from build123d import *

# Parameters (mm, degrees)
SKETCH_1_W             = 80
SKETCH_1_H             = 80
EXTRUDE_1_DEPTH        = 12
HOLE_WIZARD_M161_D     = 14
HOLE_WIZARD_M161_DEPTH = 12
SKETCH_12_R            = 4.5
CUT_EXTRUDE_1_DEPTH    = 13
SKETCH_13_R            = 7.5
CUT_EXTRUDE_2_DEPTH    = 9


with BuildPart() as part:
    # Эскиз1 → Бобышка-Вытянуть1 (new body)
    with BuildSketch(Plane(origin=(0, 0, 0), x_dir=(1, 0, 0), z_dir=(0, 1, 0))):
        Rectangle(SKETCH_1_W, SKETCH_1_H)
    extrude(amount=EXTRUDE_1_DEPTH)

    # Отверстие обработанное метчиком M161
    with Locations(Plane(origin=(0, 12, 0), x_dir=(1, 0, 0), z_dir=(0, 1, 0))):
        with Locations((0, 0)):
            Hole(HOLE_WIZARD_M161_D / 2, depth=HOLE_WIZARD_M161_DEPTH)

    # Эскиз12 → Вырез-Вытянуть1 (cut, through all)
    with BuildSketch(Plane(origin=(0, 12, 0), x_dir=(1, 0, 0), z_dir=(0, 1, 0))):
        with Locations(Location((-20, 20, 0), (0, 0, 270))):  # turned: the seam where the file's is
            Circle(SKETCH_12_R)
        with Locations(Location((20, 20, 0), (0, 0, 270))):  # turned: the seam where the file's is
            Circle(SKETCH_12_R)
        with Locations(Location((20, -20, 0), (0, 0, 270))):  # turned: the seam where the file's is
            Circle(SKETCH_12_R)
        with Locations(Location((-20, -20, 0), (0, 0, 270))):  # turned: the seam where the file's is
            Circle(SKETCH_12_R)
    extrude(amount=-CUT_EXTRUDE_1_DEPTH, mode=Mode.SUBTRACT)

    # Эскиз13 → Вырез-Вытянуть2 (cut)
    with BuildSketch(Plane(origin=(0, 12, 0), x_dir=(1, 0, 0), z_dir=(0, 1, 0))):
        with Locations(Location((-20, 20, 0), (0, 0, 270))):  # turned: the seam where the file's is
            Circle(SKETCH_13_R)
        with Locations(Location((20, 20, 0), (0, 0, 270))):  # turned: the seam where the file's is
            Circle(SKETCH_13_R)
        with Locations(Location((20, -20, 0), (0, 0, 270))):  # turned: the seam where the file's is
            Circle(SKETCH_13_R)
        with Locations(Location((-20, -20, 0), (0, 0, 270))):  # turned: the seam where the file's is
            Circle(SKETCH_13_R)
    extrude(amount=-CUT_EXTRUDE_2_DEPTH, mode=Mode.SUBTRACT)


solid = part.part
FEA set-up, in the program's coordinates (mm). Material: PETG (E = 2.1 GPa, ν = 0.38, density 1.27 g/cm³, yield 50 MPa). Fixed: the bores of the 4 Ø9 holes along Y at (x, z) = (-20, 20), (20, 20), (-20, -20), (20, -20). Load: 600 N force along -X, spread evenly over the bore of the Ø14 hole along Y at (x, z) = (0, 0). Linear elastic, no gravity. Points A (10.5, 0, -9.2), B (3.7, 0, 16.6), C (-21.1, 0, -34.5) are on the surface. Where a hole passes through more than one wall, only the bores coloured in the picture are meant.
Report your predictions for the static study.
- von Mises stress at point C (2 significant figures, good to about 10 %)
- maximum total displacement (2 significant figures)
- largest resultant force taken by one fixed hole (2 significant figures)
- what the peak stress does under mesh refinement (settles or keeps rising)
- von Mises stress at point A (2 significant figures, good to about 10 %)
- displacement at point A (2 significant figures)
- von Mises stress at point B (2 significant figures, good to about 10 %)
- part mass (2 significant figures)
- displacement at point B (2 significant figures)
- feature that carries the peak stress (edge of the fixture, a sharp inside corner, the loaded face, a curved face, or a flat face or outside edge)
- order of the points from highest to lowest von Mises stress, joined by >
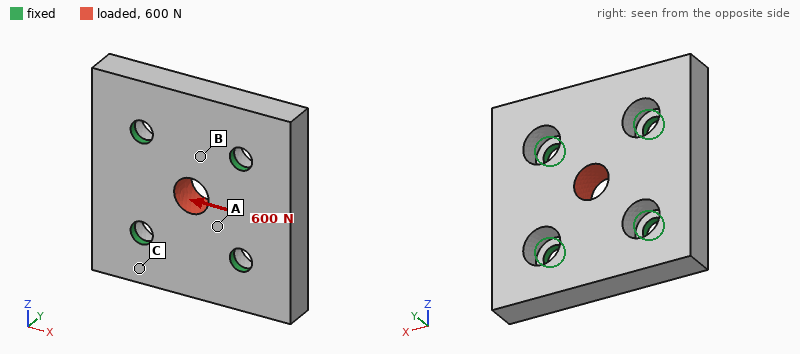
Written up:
0.35 MPa
20 µm
160 N
keeps rising
1.1 MPa
11 µm
0.76 MPa
86 g
7.8 µm
edge of the fixture
A > B > C
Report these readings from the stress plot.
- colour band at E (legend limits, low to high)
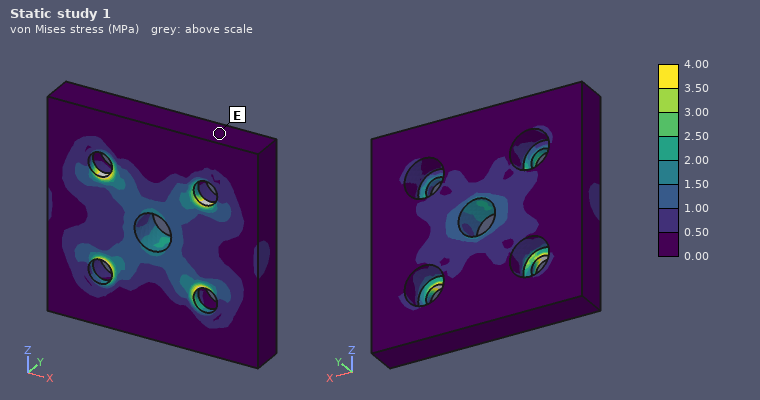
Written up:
0.00 to 0.50 MPa
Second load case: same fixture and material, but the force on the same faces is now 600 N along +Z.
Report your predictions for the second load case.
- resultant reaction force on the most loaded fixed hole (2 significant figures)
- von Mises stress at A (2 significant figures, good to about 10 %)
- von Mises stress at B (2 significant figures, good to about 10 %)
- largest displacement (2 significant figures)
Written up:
160 N
1.2 MPa
0.77 MPa
20 µm
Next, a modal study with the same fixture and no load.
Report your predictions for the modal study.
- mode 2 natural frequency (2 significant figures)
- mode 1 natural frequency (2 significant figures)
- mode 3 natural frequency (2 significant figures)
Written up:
2500 Hz
2500 Hz
2700 Hz
